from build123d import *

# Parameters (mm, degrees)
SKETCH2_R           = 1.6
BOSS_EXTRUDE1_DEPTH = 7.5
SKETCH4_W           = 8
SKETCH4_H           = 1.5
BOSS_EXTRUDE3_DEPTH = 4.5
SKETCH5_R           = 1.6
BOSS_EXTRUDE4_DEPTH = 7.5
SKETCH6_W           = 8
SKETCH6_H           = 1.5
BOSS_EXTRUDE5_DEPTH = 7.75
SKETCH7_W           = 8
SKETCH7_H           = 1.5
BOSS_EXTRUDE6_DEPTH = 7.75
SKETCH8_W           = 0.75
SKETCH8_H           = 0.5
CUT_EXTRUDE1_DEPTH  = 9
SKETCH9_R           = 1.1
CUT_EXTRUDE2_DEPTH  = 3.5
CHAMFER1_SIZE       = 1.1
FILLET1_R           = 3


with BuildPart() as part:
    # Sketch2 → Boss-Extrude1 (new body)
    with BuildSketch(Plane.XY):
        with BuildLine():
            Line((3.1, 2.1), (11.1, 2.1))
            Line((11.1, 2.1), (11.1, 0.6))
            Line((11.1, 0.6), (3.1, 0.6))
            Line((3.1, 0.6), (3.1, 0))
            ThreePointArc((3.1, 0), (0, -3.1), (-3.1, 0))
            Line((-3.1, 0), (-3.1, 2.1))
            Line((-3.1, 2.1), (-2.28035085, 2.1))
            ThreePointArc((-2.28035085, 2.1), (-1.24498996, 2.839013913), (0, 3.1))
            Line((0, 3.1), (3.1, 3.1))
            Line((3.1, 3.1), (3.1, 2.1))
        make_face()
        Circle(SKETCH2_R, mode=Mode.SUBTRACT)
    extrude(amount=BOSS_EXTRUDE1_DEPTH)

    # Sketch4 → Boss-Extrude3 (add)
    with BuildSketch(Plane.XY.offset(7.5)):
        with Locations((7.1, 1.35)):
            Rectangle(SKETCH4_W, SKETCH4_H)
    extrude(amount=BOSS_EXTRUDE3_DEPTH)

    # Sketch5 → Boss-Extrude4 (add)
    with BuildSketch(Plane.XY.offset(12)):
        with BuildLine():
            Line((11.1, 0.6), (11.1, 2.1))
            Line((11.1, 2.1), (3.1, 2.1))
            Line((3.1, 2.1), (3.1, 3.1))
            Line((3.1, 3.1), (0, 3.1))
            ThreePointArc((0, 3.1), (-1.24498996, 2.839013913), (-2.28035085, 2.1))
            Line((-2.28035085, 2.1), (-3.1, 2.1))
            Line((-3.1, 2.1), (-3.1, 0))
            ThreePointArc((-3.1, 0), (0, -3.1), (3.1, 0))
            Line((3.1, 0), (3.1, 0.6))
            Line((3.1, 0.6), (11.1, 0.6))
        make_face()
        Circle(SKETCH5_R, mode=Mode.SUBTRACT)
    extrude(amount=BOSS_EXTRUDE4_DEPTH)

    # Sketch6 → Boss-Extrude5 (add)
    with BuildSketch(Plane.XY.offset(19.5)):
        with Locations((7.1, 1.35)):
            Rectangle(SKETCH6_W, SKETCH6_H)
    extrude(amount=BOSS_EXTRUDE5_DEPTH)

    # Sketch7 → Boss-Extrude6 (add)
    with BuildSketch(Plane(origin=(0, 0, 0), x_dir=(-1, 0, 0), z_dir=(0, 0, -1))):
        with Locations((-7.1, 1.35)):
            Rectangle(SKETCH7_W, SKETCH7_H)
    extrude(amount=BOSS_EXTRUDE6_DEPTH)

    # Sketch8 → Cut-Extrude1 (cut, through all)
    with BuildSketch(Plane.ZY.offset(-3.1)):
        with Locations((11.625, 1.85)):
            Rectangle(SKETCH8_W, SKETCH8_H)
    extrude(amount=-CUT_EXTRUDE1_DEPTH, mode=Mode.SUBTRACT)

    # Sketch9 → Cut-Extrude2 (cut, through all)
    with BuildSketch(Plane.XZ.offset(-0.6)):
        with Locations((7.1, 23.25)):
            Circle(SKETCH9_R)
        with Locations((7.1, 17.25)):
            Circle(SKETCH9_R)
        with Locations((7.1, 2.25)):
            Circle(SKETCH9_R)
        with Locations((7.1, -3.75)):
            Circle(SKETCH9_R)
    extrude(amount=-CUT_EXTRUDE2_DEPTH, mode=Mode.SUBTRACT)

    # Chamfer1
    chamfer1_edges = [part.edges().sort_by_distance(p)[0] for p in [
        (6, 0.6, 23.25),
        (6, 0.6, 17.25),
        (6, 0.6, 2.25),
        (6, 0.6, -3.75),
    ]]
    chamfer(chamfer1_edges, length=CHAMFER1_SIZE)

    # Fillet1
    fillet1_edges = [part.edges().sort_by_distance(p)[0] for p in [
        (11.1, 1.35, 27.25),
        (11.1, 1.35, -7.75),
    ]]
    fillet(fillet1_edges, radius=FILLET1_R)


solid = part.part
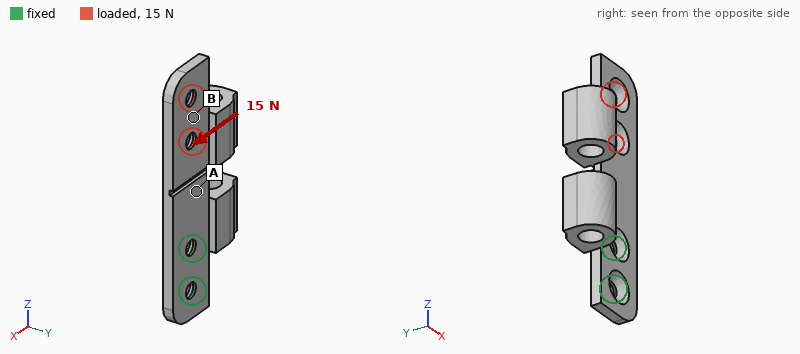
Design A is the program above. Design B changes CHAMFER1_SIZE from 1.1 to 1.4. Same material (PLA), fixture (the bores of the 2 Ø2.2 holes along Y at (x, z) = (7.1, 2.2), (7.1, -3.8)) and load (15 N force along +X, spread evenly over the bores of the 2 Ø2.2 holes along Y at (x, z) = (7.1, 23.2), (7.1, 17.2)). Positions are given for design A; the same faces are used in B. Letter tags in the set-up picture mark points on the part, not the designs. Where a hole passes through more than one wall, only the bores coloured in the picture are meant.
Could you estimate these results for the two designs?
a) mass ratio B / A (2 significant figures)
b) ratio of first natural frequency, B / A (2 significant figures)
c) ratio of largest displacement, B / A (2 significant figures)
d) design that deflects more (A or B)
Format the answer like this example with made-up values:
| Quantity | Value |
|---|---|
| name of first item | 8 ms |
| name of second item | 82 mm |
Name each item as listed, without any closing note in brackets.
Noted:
| Quantity | Value |
|---|---|
| mass ratio B / A | 0.98 |
| ratio of first natural frequency, B / A | 0.95 |
| ratio of largest displacement, B / A | 1.2 |
| design that deflects more | B |
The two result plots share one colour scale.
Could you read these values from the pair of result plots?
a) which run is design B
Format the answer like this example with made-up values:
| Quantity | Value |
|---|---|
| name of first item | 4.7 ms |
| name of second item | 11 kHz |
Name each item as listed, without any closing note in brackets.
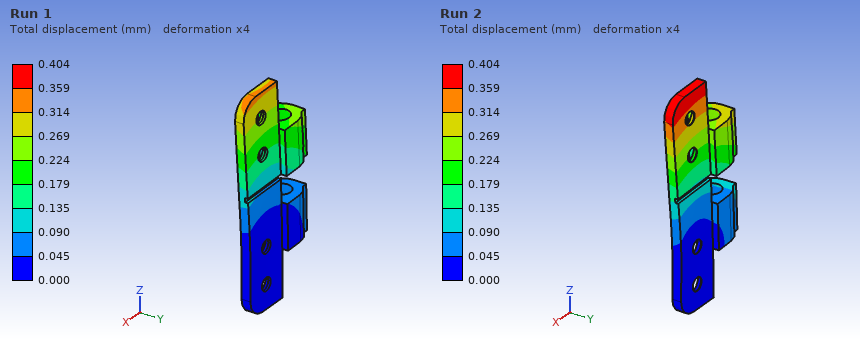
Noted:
| Quantity | Value |
|---|---|
| which run is design B | Run 2 |
